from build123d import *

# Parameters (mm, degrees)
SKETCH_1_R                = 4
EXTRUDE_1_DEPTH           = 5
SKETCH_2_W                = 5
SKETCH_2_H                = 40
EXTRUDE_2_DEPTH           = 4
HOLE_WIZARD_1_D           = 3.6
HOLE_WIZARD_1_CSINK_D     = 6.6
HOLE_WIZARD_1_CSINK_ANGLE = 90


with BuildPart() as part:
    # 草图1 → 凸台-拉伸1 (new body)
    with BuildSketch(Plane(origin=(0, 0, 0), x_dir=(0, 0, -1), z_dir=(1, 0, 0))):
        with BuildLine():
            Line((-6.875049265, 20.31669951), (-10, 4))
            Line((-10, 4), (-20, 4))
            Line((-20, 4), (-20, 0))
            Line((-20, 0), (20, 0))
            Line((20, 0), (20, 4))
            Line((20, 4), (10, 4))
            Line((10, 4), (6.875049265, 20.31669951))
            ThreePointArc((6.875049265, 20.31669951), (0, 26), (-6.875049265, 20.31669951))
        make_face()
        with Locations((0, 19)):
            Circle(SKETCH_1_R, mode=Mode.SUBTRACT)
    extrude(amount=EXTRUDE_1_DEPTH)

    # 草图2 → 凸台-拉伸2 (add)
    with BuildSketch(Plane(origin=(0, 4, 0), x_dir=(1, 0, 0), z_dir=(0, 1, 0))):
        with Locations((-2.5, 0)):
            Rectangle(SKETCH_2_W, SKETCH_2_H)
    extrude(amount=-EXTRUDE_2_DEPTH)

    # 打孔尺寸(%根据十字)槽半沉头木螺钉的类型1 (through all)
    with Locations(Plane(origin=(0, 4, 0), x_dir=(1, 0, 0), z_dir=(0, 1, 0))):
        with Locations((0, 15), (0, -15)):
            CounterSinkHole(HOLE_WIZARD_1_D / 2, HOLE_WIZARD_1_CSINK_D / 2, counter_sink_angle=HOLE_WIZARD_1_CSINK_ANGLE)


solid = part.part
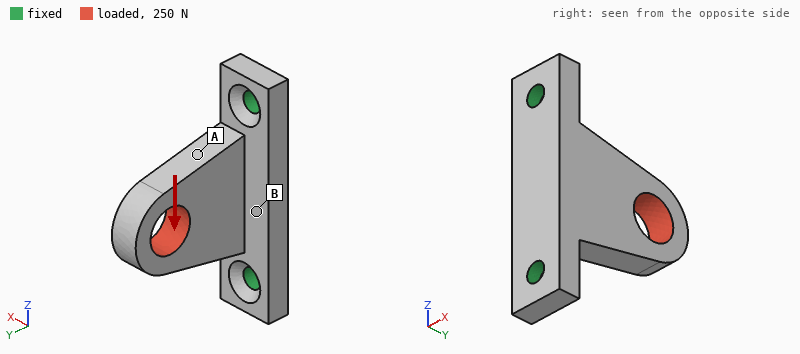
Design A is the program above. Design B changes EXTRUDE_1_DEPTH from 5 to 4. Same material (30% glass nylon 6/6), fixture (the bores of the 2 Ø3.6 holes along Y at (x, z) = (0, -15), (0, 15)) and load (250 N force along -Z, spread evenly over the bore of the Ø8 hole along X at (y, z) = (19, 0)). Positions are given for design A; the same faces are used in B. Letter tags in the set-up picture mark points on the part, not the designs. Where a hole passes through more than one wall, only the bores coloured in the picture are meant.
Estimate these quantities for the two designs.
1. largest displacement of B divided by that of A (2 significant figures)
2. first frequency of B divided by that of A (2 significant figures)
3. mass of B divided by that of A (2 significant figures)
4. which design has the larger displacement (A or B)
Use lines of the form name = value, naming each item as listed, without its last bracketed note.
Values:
largest displacement of B divided by that of A = 1.2
first frequency of B divided by that of A = 0.97
mass of B divided by that of A = 0.85
which design has the larger displacement = B
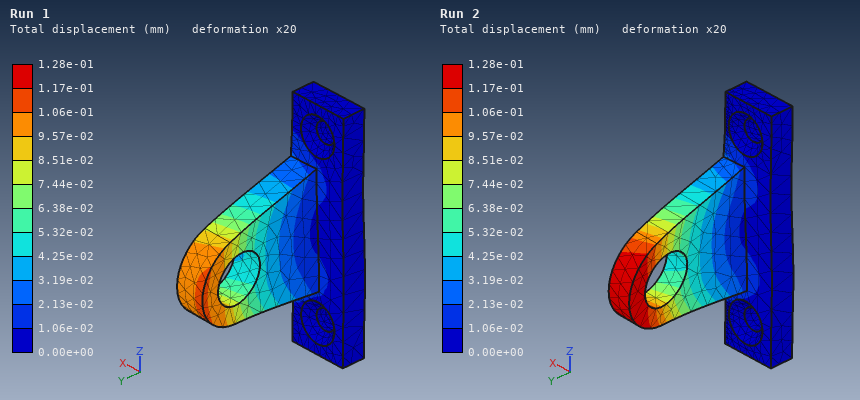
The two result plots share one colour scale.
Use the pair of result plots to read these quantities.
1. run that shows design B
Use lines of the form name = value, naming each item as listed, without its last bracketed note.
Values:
run that shows design B = Run 2
